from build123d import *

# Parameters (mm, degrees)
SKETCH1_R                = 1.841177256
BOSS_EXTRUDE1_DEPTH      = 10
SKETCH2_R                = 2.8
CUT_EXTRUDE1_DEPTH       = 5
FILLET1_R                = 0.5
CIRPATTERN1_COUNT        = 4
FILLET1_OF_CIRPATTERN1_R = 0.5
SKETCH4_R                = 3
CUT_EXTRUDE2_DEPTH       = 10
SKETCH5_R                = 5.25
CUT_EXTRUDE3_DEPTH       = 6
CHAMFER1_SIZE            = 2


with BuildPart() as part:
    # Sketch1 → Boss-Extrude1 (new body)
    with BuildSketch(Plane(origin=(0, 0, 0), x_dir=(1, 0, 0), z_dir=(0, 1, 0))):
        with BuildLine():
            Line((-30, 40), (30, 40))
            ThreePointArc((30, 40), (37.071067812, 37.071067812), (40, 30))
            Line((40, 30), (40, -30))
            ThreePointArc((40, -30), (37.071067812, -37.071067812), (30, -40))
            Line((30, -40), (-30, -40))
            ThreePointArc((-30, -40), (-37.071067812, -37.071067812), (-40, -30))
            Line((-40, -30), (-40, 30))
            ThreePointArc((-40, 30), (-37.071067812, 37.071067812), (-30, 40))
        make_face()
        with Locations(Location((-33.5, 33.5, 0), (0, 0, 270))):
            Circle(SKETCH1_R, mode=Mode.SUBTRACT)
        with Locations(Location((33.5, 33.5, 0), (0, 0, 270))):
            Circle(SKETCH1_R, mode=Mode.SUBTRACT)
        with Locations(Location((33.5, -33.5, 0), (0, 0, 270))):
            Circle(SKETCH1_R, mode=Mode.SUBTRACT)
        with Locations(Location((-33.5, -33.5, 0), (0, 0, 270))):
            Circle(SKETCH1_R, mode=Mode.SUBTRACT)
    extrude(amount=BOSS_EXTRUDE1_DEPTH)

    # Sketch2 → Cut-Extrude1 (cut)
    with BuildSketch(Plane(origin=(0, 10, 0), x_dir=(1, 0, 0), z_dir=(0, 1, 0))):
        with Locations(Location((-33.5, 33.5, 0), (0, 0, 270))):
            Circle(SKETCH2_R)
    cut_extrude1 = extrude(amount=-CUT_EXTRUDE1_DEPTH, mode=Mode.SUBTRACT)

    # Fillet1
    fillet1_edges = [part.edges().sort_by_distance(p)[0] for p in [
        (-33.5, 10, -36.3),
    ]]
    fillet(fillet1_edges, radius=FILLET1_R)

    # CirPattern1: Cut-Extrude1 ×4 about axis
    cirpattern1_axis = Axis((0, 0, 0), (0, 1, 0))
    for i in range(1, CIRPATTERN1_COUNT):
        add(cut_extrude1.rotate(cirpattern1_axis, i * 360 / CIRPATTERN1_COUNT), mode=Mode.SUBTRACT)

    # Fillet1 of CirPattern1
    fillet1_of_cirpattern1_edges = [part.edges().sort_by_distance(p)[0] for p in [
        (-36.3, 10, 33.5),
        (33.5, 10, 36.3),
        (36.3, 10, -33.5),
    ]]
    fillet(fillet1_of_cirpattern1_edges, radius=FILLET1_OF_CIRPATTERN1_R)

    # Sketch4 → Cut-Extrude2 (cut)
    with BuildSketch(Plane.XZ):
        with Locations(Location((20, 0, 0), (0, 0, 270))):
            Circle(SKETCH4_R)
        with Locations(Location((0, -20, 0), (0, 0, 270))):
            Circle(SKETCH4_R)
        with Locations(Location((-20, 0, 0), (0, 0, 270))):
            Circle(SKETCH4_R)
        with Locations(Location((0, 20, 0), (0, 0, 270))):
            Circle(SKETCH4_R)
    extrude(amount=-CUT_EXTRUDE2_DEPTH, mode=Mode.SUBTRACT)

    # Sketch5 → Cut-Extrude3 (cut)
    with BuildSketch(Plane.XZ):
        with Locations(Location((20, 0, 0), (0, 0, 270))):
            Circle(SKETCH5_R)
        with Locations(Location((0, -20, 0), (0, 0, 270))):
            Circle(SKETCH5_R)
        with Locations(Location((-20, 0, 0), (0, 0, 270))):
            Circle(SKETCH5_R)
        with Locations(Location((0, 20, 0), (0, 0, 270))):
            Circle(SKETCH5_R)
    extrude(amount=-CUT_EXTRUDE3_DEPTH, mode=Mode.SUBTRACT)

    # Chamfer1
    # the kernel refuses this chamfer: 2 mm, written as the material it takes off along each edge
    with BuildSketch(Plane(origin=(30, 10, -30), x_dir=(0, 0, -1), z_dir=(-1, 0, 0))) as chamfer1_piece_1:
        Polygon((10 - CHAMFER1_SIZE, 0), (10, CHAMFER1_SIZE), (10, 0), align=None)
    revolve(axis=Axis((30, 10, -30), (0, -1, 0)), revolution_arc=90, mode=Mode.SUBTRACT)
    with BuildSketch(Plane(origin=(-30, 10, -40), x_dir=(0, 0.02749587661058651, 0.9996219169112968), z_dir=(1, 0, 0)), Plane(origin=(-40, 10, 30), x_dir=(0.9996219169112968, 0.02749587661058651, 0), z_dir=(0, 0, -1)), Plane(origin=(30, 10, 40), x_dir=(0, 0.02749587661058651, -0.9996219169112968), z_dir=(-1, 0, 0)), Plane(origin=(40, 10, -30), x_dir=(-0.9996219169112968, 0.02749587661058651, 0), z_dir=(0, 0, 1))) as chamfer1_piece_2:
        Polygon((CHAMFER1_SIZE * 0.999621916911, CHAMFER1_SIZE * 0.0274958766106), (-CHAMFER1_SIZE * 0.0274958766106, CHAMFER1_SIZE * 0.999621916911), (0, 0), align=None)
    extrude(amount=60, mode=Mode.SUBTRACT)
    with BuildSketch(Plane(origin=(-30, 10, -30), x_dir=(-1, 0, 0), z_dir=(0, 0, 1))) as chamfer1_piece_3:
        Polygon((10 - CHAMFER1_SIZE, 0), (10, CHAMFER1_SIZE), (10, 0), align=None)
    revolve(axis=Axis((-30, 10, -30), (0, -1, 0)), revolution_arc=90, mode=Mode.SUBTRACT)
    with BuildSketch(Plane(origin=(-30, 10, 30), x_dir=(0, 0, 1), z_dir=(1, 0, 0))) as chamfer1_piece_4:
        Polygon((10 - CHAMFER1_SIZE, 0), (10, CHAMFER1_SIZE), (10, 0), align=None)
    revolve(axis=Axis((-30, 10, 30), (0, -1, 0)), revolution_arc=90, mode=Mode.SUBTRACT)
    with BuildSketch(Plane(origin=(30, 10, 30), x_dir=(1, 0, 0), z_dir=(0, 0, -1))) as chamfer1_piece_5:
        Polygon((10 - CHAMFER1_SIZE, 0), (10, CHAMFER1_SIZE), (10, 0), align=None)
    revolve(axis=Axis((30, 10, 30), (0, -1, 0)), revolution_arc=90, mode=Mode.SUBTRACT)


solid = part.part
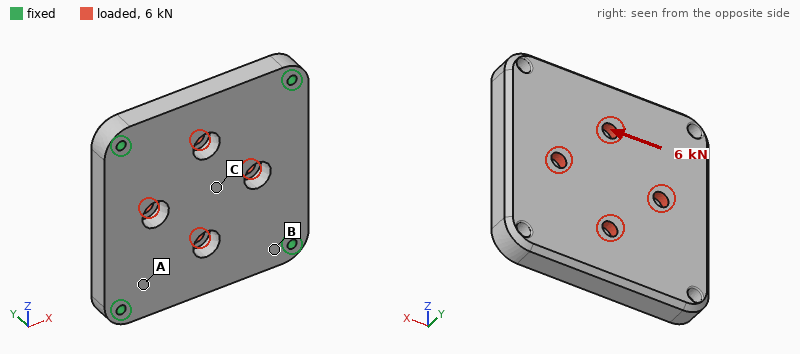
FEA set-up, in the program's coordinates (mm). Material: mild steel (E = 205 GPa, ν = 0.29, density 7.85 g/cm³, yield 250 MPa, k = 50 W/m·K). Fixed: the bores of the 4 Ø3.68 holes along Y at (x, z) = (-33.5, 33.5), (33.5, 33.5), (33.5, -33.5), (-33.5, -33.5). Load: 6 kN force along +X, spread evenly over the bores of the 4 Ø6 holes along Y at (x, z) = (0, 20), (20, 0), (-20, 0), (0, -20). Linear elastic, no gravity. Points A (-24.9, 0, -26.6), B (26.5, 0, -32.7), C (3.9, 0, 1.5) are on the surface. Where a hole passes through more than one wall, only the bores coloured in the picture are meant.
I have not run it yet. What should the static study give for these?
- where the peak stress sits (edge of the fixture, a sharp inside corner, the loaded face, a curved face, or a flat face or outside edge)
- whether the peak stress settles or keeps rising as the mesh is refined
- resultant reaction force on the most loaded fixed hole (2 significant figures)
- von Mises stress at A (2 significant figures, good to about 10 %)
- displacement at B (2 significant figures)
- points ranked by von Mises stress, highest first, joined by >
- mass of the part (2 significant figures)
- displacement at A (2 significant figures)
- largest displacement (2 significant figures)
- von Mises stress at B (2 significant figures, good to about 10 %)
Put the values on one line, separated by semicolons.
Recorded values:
edge of the fixture; keeps rising; 1.6 kN; 12 MPa; 0.57 µm; B > A > C; 470 g; 1.1 µm; 3.1 µm; 18 MPa
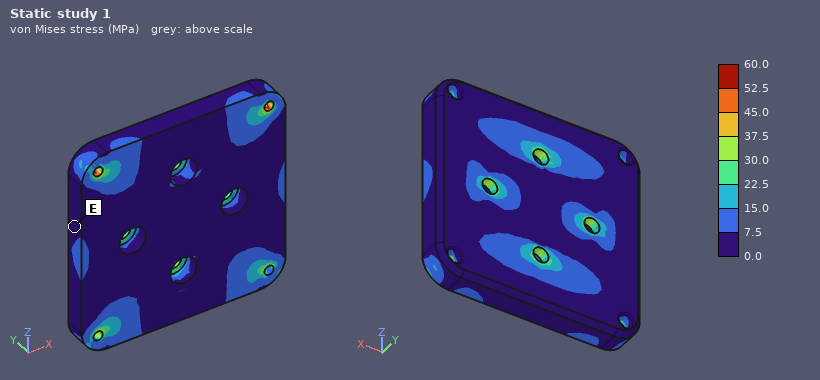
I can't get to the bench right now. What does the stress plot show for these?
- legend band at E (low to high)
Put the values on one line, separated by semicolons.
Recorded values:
0.0 to 7.5 MPa
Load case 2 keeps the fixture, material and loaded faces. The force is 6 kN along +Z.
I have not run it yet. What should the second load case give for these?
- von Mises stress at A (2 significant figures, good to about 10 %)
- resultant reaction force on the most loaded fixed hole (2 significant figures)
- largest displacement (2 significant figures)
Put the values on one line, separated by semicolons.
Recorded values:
11 MPa; 1.6 kN; 3.1 µm
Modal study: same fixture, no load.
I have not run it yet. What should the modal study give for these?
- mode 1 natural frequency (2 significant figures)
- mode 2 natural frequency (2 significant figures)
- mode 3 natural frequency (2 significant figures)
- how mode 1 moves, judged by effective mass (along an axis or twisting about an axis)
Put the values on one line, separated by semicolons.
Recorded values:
5300 Hz; 8900 Hz; 8900 Hz; along Y
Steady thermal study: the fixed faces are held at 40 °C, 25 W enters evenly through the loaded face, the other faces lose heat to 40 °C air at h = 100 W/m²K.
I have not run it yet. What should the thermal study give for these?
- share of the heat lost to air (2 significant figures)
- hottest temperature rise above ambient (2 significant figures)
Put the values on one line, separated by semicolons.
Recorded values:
44 %; 15 K
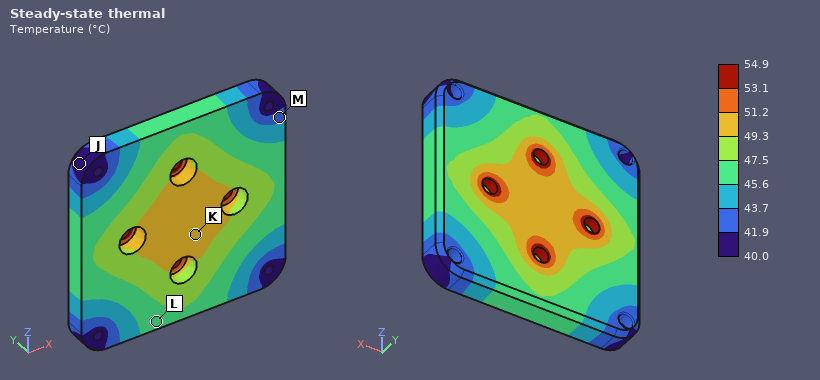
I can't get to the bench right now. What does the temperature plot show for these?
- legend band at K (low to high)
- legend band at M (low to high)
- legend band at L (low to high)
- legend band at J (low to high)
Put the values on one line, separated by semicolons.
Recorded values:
49.3 to 51.2 °C; 41.9 to 43.7 °C; 45.6 to 47.5 °C; 40.0 to 41.9 °C
